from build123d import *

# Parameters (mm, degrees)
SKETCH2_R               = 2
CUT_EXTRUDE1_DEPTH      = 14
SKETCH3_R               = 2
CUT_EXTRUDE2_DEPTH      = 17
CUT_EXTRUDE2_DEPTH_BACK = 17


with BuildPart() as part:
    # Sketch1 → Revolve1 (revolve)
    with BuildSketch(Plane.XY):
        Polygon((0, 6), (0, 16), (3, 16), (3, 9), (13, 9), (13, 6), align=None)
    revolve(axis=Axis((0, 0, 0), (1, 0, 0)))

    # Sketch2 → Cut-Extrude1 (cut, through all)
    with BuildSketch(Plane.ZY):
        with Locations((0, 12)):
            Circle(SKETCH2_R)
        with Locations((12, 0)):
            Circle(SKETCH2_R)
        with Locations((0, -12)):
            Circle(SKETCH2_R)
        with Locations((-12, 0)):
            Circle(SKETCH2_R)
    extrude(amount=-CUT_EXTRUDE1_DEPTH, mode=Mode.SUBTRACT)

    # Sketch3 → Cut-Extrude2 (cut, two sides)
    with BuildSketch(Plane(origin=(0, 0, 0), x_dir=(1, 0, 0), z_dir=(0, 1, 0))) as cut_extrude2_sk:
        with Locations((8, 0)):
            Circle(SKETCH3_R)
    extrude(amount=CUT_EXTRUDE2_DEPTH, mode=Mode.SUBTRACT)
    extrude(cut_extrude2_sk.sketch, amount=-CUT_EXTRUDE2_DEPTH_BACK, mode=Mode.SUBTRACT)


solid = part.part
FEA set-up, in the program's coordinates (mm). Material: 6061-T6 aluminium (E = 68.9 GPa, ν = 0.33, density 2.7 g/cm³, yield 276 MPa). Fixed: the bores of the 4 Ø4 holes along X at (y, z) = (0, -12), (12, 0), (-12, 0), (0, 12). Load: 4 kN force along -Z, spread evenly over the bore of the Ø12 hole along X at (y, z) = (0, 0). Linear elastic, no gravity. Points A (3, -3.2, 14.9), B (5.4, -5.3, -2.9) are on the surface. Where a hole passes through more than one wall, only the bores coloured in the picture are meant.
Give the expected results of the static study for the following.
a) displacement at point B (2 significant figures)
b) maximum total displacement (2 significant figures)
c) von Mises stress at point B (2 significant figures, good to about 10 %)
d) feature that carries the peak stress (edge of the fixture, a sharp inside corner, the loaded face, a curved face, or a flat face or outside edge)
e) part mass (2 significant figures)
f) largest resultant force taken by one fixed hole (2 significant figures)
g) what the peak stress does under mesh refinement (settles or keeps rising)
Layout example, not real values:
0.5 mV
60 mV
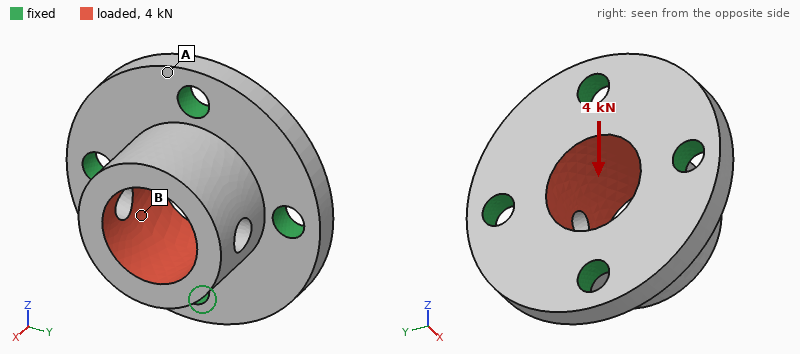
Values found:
8.3 µm
23 µm
43 MPa
edge of the fixture
8.8 g
1.5 kN
keeps rising
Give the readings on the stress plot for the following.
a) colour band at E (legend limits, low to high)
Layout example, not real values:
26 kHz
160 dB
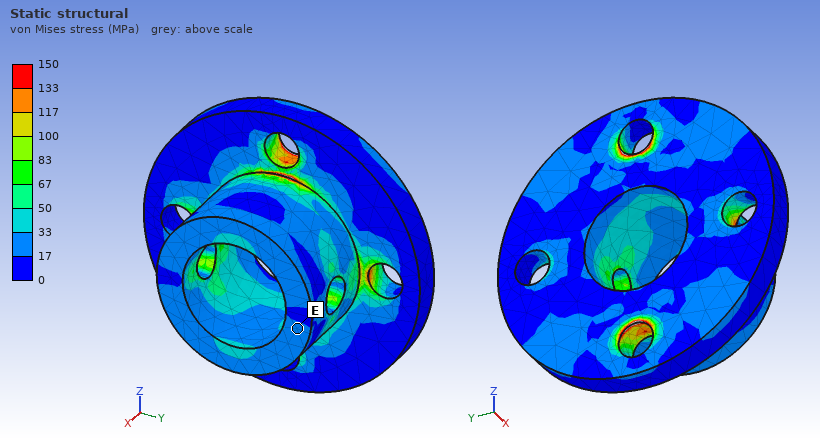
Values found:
17 to 33 MPa
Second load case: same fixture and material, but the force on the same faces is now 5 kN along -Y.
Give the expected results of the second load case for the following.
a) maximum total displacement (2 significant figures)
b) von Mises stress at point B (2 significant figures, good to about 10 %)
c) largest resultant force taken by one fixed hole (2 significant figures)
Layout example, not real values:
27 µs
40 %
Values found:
27 µm
44 MPa
1.8 kN
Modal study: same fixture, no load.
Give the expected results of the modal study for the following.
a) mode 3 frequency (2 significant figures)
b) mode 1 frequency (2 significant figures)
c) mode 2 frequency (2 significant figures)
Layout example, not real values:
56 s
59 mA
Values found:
38 kHz
34 kHz
35 kHz
